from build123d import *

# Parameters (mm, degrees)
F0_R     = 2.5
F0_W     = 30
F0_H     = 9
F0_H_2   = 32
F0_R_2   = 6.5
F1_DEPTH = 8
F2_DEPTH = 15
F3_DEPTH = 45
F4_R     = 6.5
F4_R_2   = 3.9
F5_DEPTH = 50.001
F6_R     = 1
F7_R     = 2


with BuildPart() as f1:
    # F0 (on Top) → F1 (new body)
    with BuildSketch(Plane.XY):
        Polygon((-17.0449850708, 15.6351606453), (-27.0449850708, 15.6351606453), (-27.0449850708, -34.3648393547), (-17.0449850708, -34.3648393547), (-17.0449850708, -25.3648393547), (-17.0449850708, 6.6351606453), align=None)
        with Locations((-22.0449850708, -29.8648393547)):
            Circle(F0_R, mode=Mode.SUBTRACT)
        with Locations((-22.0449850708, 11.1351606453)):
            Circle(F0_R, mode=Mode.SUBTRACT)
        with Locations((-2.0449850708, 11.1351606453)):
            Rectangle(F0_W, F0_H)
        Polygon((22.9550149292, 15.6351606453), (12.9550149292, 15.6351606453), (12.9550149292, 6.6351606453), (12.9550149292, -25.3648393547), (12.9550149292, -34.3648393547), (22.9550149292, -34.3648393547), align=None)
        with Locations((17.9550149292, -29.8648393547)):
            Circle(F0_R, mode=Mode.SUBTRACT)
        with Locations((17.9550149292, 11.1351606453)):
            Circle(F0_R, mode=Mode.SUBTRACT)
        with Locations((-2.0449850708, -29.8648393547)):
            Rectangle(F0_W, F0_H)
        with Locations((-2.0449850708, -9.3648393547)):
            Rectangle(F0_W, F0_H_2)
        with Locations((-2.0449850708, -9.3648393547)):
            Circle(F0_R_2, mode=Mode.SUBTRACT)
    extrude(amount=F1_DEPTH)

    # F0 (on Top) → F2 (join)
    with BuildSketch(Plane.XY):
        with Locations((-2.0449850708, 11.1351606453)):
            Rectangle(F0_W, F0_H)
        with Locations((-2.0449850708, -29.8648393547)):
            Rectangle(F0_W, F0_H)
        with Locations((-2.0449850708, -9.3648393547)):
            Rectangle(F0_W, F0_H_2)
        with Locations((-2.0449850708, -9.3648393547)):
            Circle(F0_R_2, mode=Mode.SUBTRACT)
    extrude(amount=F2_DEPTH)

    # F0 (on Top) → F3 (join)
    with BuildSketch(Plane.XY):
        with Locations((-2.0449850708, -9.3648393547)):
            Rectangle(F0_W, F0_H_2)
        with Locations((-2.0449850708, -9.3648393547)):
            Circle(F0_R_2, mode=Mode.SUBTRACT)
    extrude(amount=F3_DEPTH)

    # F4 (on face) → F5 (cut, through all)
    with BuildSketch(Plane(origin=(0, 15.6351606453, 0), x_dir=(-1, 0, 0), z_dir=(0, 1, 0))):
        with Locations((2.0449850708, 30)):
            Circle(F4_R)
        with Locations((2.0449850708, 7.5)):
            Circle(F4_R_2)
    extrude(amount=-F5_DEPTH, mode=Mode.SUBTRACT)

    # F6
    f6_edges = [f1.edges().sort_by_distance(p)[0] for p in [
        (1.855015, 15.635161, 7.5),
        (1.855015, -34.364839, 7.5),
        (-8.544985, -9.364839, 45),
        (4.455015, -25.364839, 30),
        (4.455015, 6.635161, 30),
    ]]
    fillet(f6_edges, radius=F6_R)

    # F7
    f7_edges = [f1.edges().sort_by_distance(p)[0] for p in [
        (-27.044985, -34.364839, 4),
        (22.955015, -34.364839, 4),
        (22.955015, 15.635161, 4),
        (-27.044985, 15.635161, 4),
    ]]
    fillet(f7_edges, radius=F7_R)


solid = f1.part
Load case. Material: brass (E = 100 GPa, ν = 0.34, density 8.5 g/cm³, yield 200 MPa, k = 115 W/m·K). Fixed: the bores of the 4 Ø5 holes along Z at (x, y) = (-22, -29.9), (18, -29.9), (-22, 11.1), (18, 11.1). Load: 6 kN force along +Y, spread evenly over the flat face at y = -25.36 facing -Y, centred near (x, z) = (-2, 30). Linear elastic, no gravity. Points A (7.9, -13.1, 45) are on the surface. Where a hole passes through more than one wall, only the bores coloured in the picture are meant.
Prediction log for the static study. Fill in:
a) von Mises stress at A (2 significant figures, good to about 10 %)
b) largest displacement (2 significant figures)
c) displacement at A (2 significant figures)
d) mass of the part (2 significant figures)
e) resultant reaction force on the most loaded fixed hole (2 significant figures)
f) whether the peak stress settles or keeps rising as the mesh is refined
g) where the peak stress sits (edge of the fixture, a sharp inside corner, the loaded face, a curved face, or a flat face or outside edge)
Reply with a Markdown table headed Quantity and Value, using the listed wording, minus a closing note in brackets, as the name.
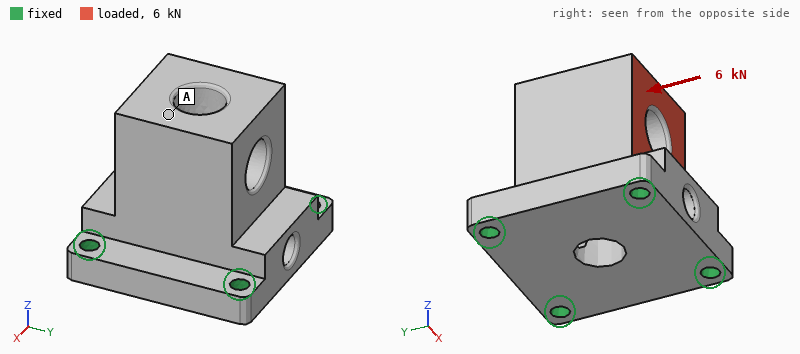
| Quantity | Value |
|---|---|
| von Mises stress at A | 9.6 MPa |
| largest displacement | 28 µm |
| displacement at A | 25 µm |
| mass of the part | 410 g |
| resultant reaction force on the most loaded fixed hole | 2.7 kN |
| whether the peak stress settles or keeps rising as the mesh is refined | keeps rising |
| where the peak stress sits | edge of the fixture |
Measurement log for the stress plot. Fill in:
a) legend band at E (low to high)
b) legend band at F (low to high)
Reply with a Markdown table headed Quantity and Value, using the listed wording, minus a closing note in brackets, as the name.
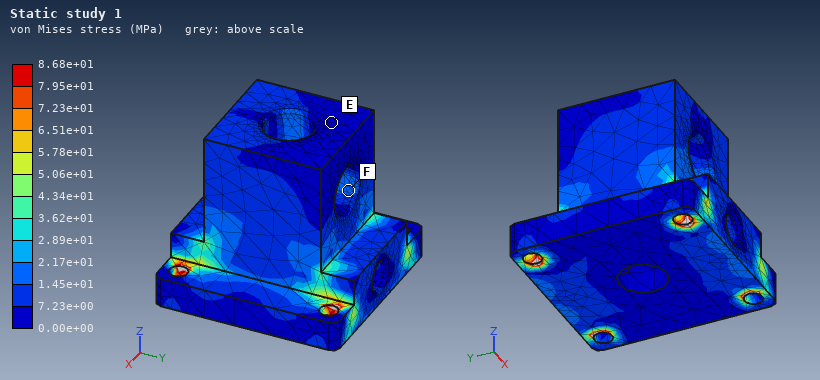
| Quantity | Value |
|---|---|
| legend band at E | 0.00e+00 to 7.23e+00 MPa |
| legend band at F | 1.45e+01 to 2.17e+01 MPa |
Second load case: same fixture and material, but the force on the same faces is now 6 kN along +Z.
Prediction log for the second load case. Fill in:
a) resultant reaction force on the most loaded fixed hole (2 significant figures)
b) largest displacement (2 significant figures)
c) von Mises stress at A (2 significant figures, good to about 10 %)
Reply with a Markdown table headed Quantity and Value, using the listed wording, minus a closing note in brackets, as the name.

| Quantity | Value |
|---|---|
| resultant reaction force on the most loaded fixed hole | 2.9 kN |
| largest displacement | 26 µm |
| von Mises stress at A | 14 MPa |
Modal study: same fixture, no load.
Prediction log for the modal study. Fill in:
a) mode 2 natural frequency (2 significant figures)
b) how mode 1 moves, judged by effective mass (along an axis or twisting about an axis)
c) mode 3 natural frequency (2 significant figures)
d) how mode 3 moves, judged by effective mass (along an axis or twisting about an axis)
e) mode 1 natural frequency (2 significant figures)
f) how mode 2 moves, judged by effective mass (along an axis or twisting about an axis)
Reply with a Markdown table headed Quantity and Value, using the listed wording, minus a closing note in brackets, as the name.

| Quantity | Value |
|---|---|
| mode 2 natural frequency | 6200 Hz |
| how mode 1 moves, judged by effective mass | along X |
| mode 3 natural frequency | 8700 Hz |
| how mode 3 moves, judged by effective mass | along Z |
| mode 1 natural frequency | 5400 Hz |
| how mode 2 moves, judged by effective mass | along Y |
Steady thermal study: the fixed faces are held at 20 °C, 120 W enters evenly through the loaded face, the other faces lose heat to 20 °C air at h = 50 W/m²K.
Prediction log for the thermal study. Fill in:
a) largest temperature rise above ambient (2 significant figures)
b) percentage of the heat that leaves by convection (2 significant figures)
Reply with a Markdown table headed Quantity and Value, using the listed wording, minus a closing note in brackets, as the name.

| Quantity | Value |
|---|---|
| largest temperature rise above ambient | 63 K |
| percentage of the heat that leaves by convection | 13 % |
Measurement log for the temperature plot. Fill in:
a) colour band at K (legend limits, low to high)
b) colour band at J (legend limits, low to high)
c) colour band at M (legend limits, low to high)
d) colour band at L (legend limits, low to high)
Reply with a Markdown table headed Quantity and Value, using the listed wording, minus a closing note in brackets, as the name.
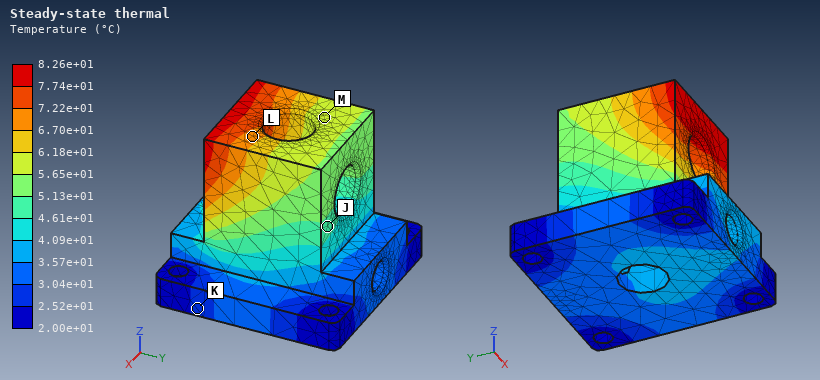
| Quantity | Value |
|---|---|
| colour band at K | 2.52e+01 to 3.04e+01 °C |
| colour band at J | 4.61e+01 to 5.13e+01 °C |
| colour band at M | 5.65e+01 to 6.18e+01 °C |
| colour band at L | 6.70e+01 to 7.22e+01 °C |
